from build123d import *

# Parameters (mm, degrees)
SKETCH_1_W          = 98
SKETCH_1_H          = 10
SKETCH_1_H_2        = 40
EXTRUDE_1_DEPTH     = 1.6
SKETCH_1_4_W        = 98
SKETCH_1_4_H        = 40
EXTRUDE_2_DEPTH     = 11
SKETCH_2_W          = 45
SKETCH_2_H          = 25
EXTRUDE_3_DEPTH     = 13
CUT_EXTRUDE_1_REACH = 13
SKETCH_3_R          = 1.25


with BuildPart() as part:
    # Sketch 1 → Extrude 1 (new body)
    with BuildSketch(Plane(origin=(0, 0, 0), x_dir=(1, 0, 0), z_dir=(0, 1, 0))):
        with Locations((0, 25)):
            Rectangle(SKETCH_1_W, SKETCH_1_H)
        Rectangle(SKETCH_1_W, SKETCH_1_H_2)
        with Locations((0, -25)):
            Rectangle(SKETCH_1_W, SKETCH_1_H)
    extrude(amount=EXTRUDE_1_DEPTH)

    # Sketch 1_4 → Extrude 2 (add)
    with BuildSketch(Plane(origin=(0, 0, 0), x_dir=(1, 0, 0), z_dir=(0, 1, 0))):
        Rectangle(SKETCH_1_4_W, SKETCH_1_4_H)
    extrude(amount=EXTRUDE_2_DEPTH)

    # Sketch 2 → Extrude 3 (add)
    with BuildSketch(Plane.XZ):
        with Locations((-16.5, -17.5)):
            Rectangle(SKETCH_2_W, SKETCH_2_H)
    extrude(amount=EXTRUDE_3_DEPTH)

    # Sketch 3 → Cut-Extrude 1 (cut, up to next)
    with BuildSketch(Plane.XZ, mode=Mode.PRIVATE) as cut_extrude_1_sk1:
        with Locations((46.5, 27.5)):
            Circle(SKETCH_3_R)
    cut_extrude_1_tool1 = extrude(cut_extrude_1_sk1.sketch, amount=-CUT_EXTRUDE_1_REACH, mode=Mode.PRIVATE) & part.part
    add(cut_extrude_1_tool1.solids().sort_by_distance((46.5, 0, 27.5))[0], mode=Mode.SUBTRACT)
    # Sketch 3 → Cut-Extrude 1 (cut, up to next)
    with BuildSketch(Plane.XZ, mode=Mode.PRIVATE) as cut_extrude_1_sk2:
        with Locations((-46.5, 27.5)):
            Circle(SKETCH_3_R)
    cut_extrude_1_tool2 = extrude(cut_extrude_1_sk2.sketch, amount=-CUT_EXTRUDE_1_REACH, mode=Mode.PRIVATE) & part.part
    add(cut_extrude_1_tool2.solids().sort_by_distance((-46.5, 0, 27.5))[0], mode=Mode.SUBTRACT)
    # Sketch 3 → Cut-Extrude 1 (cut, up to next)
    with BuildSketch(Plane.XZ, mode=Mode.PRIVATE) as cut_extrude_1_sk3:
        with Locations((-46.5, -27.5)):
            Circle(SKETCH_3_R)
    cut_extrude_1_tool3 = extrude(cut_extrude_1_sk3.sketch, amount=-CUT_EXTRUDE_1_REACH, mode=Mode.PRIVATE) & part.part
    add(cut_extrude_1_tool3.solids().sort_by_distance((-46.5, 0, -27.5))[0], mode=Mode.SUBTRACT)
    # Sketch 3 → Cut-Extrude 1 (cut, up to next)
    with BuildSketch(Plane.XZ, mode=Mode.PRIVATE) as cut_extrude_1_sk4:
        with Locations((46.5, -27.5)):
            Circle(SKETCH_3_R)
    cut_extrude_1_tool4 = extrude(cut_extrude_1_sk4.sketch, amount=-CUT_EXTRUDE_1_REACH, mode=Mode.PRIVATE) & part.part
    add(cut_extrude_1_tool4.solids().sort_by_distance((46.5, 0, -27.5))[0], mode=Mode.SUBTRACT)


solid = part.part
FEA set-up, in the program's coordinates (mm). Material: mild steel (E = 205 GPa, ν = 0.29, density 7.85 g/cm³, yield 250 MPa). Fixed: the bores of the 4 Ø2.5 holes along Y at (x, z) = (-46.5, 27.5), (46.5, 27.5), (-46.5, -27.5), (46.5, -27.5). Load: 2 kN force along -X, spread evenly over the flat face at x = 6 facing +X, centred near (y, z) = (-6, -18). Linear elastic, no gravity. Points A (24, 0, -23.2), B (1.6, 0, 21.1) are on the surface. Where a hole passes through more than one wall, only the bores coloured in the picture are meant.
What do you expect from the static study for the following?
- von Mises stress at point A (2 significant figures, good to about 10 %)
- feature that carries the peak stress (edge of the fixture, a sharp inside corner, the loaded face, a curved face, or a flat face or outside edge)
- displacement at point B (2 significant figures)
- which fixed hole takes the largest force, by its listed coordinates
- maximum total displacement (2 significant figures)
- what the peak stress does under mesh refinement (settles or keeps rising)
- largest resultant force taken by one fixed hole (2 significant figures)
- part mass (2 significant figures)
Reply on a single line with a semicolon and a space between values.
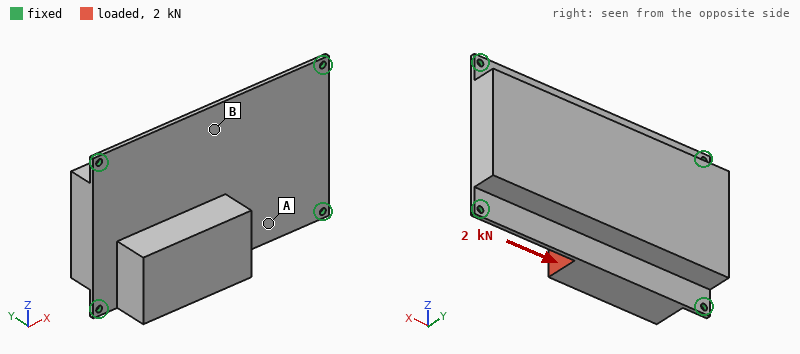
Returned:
16 MPa; edge of the fixture; 3.9 µm; (-46.5, -27.5); 12 µm; keeps rising; 830 N; 480 g
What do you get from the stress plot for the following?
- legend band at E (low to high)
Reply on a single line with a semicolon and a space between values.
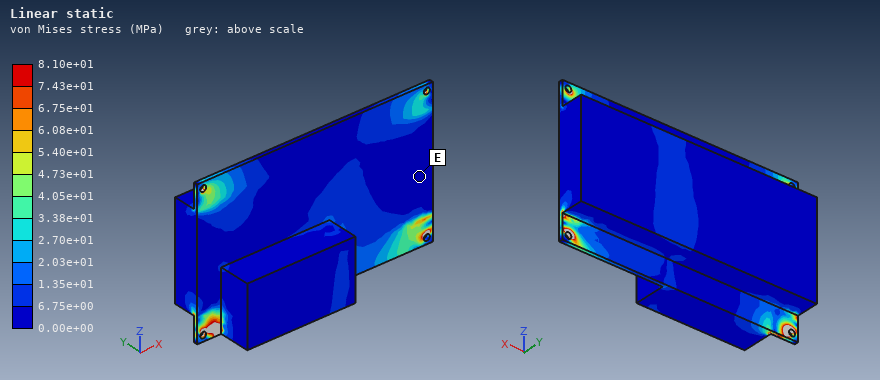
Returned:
0.00e+00 to 6.75e+00 MPa
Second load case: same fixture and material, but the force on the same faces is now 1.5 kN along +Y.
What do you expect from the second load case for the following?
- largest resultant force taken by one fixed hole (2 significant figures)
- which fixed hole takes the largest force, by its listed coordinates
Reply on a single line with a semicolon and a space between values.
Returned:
760 N; (46.5, -27.5)
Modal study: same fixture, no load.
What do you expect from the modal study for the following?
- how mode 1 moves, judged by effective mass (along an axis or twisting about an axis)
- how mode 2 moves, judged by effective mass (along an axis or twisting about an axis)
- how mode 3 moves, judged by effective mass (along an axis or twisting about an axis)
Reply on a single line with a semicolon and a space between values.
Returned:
along Y; twisting about X; twisting about Z
